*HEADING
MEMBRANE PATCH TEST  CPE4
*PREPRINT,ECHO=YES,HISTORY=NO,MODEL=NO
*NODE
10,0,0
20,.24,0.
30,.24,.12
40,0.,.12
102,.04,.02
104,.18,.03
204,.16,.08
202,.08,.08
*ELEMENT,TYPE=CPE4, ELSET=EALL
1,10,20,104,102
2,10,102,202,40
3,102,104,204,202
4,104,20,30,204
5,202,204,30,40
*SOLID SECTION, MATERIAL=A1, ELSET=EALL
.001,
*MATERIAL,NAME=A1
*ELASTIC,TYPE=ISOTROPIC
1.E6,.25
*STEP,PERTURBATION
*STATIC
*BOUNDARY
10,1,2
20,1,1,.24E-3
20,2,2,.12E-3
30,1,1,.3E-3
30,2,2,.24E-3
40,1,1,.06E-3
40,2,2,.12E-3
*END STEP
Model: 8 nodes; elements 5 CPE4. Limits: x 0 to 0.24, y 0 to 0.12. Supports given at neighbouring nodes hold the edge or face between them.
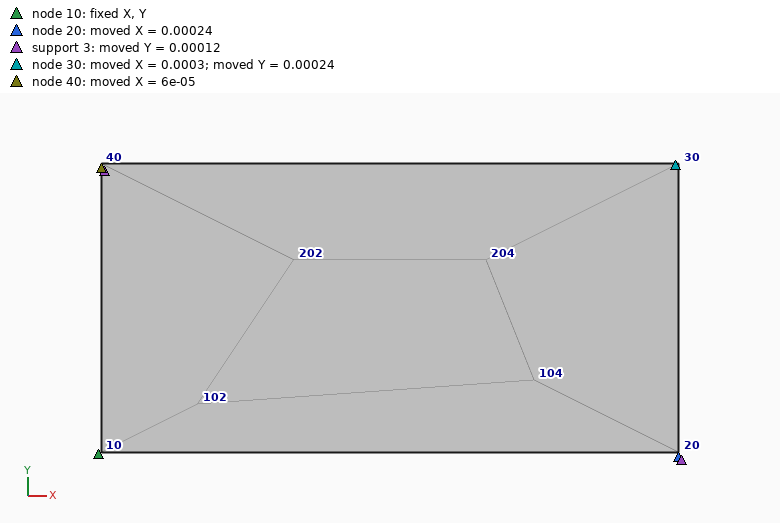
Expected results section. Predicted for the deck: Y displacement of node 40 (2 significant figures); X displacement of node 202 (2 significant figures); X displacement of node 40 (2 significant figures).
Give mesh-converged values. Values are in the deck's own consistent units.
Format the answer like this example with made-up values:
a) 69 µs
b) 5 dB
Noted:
a) 1.2e-04
b) 1.2e-04
c) 6.0e-05
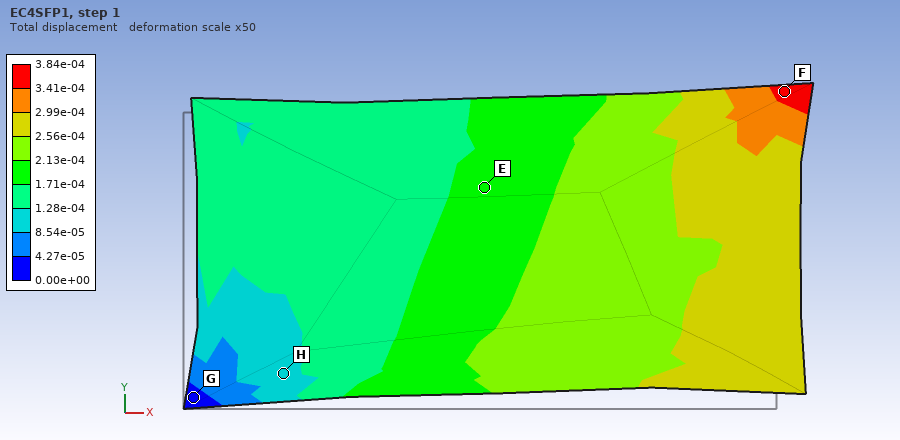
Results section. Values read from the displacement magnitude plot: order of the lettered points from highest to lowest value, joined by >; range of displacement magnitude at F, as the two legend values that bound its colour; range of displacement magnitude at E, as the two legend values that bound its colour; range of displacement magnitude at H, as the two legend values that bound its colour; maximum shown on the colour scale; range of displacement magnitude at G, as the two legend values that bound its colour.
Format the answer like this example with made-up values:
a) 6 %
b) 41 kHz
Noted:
a) F > E > H > G
b) 3.41e-04 to 3.84e-04
c) 1.71e-04 to 2.13e-04
d) 8.54e-05 to 1.28e-04
e) 3.84e-04
f) 0.00e+00 to 4.27e-05
